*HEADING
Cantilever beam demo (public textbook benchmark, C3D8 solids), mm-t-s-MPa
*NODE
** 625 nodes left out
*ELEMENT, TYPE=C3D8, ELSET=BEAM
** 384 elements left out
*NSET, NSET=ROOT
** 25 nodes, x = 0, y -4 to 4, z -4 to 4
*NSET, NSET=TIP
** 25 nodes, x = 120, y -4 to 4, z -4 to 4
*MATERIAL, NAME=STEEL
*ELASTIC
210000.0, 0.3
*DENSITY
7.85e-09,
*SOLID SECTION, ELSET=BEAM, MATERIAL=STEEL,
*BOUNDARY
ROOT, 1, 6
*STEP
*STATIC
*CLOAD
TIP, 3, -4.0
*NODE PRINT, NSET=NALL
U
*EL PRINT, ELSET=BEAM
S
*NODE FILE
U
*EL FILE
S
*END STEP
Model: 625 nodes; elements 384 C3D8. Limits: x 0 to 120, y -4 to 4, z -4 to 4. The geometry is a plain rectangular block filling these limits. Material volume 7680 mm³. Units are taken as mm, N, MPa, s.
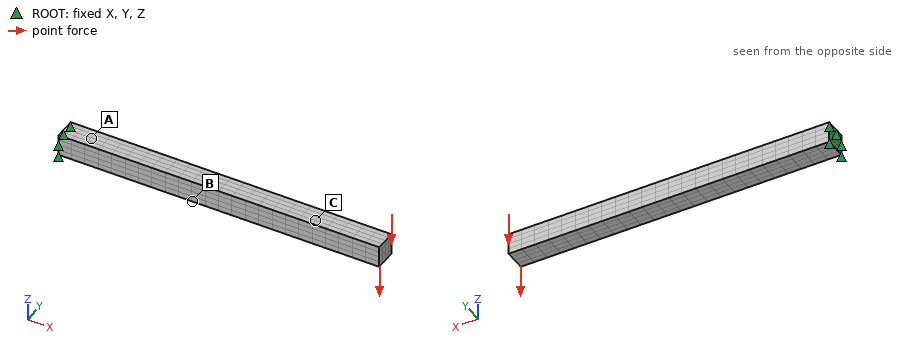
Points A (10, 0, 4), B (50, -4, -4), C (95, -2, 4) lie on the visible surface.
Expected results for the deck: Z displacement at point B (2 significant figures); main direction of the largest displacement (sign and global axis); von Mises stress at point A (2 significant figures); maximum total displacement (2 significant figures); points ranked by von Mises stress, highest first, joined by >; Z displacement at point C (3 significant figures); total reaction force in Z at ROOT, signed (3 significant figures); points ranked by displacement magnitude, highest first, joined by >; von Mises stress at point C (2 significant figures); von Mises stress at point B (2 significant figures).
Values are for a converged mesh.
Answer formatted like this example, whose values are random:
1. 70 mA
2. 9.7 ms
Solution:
1. -0.18 mm
2. -Z
3. 130 MPa
4. 0.80 mm
5. A > B > C
6. -0.555 mm
7. 100 N
8. C > B > A
9. 29 MPa
10. 82 MPa
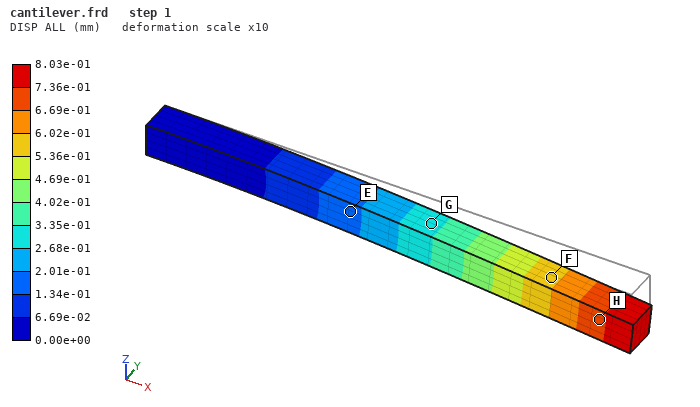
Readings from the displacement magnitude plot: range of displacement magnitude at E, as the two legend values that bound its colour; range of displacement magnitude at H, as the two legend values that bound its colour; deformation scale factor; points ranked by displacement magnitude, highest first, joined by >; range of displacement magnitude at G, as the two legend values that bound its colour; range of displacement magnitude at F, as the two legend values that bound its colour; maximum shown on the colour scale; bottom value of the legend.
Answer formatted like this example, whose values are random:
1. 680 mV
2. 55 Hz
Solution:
1. 1.34e-01 to 2.01e-01 mm
2. 6.69e-01 to 7.36e-01 mm
3. 10
4. H > F > G > E
5. 2.68e-01 to 3.35e-01 mm
6. 5.36e-01 to 6.02e-01 mm
7. 8.03e-01 mm
8. 0.00e+00 mm
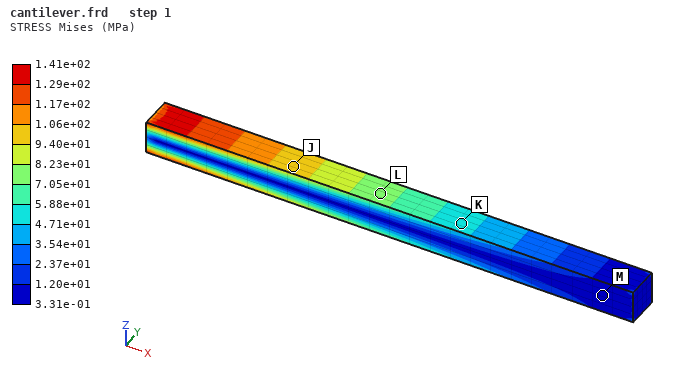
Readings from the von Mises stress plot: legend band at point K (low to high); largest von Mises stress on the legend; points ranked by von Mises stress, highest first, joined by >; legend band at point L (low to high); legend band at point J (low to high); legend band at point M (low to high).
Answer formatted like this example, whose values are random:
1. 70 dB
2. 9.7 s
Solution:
1. 4.71e+01 to 5.88e+01 MPa
2. 1.41e+02 MPa
3. J > L > K > M
4. 7.05e+01 to 8.23e+01 MPa
5. 9.40e+01 to 1.06e+02 MPa
6. 3.31e-01 to 1.20e+01 MPa
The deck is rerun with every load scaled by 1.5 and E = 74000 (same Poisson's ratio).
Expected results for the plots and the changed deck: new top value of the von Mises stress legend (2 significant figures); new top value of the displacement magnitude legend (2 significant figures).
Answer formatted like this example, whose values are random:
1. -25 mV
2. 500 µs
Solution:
1. 210 MPa
2. 3.4 mm
